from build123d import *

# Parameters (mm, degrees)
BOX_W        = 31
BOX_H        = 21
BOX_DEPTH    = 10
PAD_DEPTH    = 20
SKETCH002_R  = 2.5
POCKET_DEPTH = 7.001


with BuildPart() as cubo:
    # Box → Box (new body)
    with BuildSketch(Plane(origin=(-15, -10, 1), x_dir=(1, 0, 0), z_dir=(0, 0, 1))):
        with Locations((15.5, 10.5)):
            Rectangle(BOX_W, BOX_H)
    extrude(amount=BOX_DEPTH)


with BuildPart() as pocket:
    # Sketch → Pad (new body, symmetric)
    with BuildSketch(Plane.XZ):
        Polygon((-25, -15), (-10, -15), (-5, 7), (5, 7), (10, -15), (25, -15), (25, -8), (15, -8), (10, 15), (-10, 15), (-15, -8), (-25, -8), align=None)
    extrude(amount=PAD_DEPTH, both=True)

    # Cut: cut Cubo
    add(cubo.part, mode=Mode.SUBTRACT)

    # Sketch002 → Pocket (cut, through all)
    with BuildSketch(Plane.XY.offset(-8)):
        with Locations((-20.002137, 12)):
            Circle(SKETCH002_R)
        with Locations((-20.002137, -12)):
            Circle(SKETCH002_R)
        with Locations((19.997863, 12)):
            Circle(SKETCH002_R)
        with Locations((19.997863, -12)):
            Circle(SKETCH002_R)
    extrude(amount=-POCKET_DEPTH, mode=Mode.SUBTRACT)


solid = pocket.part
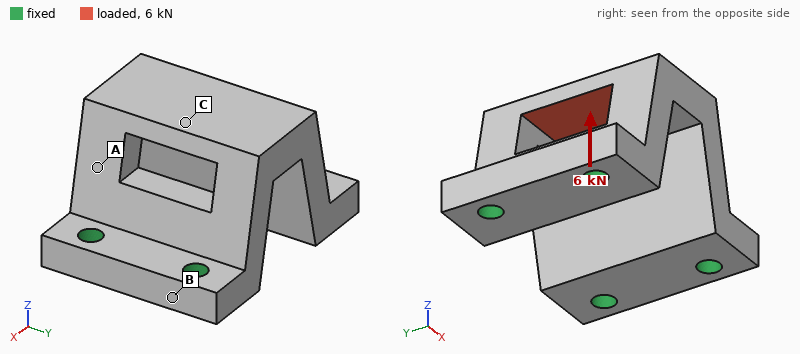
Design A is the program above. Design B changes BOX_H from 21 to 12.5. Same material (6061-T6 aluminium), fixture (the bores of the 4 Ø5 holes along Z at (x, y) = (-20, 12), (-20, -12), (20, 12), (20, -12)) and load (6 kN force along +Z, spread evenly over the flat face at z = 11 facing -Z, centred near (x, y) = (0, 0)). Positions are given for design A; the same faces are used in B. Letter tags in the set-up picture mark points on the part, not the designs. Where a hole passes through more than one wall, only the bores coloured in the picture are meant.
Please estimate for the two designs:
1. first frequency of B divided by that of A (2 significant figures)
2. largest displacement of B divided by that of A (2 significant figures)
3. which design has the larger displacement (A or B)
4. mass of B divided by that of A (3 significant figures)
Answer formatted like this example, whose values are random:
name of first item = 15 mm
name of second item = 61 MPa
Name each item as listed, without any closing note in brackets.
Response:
first frequency of B divided by that of A = 1.1
largest displacement of B divided by that of A = 0.49
which design has the larger displacement = A
mass of B divided by that of A = 1.07
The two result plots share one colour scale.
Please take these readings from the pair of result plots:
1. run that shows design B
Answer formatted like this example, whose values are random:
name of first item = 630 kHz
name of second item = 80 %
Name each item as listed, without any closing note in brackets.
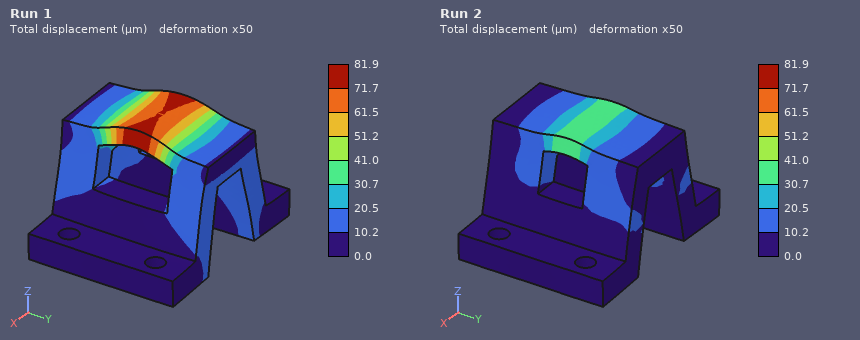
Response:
run that shows design B = Run 2
